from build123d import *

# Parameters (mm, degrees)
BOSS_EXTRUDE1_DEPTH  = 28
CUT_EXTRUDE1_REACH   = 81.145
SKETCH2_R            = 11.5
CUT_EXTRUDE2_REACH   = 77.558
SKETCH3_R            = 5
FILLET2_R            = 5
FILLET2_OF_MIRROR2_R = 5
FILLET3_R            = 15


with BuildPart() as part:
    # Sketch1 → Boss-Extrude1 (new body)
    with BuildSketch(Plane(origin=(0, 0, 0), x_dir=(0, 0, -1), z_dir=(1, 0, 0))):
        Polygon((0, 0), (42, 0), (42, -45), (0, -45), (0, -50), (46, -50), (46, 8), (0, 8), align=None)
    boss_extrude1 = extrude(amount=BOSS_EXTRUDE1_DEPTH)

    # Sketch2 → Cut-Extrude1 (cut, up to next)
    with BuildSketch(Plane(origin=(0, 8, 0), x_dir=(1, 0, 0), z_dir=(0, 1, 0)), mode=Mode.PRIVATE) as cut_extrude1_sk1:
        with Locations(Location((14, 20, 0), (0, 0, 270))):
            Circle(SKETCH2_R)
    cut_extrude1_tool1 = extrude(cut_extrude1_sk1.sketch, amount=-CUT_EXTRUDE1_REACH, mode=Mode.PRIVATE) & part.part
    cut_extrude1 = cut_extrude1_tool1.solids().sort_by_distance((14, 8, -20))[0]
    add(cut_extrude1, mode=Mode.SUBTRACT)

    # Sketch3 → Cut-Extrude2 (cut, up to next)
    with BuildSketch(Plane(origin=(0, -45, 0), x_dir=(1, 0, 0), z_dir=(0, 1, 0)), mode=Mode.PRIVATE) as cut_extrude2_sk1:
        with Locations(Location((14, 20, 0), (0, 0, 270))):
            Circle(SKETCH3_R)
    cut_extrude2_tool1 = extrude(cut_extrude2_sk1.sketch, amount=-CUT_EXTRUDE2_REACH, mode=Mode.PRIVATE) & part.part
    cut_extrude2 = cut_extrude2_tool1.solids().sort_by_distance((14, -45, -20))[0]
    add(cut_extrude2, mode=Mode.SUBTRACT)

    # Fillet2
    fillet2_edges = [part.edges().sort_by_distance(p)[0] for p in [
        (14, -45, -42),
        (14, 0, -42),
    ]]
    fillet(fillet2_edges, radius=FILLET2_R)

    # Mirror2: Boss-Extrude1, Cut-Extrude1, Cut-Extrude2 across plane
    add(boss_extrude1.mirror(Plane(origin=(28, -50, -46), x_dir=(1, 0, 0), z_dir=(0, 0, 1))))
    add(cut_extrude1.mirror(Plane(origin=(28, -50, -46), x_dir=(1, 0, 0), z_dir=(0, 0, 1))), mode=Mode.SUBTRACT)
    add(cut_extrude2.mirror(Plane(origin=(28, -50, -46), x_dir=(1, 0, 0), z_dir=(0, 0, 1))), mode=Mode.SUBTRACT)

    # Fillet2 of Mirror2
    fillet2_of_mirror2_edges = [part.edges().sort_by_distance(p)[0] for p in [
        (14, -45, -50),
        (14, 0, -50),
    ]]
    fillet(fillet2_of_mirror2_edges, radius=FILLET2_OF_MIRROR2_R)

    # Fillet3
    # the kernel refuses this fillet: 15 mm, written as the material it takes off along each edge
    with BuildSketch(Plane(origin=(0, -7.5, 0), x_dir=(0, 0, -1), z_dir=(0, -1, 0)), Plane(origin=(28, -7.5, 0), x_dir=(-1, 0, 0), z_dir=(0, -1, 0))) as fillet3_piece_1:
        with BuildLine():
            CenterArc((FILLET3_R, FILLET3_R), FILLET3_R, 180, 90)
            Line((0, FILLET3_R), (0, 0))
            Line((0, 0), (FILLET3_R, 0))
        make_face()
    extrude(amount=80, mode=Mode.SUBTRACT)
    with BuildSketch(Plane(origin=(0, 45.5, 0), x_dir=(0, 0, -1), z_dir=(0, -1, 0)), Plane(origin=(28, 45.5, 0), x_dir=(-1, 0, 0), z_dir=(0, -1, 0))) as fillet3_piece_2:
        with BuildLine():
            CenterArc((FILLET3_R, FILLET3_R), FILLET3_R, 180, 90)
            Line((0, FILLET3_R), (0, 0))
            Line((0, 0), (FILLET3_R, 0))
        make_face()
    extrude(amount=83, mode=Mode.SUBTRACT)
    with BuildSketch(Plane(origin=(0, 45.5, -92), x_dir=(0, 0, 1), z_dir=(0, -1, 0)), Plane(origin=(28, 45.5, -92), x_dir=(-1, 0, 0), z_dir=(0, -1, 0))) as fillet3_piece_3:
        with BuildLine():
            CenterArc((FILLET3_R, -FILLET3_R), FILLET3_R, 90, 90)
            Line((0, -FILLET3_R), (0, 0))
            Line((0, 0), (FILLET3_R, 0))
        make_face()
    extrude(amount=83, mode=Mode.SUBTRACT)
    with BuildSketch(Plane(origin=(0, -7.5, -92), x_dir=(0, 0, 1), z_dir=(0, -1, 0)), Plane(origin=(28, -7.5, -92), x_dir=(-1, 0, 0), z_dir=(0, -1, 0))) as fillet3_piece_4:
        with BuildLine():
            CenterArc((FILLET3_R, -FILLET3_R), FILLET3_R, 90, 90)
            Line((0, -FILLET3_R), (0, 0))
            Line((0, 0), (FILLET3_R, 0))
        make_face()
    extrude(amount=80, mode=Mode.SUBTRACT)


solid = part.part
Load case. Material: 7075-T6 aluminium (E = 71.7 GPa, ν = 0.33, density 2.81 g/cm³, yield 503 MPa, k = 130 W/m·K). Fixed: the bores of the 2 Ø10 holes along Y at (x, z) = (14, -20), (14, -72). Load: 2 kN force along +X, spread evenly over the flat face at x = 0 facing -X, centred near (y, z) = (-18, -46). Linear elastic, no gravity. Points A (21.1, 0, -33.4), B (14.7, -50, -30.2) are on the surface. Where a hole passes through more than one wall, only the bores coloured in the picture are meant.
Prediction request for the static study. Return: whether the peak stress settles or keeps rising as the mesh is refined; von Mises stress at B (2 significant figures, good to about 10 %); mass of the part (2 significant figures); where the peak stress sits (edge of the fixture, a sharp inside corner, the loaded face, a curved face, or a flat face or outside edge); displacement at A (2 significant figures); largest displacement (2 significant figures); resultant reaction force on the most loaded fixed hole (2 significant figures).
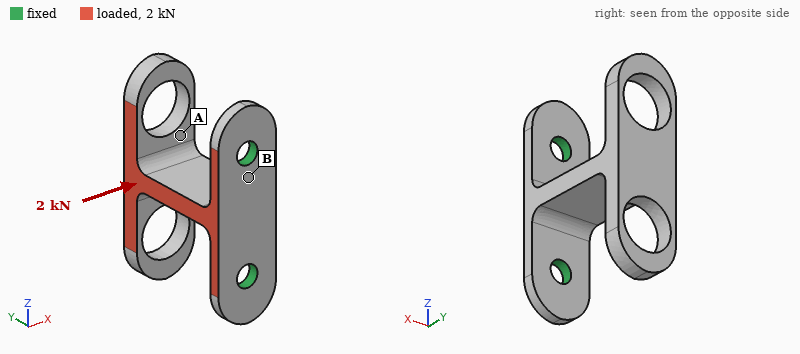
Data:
keeps rising
140 MPa
96 g
edge of the fixture
0.62 mm
0.76 mm
1.0 kN
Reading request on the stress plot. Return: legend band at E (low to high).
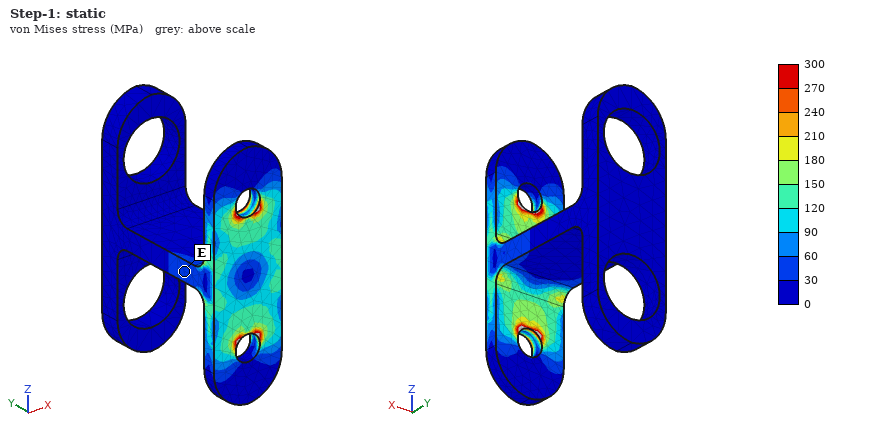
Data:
30 to 60 MPa
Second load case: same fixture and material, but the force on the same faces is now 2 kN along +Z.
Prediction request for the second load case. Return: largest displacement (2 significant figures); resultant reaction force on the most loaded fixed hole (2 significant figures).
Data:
1.1 mm
2.1 kN
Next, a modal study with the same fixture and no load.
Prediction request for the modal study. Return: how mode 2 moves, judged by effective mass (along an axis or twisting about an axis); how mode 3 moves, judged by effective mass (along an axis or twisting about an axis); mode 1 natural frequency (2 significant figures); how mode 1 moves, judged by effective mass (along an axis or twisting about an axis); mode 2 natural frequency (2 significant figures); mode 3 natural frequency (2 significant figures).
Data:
along X
twisting about Y
850 Hz
along Z
970 Hz
1700 Hz
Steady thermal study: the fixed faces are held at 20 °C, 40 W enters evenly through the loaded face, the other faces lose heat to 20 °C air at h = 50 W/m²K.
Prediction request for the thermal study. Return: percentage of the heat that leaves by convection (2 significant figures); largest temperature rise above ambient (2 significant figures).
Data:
32 %
38 K
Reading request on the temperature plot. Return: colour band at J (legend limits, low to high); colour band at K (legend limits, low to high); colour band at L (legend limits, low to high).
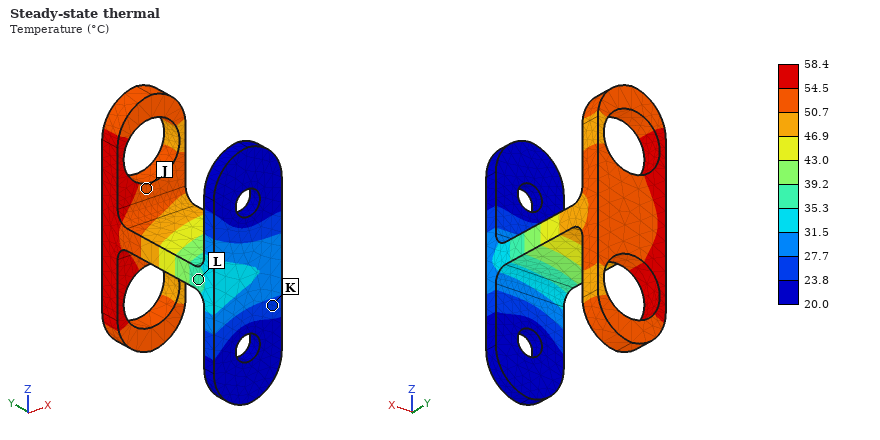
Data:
50.7 to 54.5 °C
23.8 to 27.7 °C
35.3 to 39.2 °C
